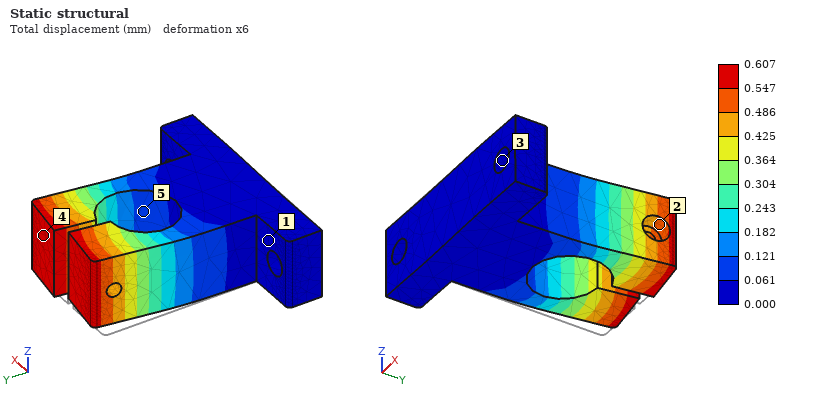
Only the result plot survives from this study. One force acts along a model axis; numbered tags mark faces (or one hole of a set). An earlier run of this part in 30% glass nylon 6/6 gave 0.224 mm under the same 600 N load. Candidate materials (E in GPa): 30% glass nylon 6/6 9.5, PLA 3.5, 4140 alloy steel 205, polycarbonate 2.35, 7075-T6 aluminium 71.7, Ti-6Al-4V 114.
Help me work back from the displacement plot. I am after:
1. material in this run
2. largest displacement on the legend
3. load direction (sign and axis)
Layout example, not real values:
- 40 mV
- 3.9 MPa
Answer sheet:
- PLA
- 0.607 mm
- +X
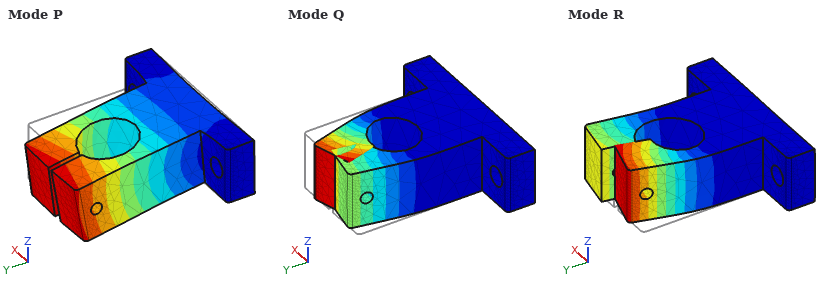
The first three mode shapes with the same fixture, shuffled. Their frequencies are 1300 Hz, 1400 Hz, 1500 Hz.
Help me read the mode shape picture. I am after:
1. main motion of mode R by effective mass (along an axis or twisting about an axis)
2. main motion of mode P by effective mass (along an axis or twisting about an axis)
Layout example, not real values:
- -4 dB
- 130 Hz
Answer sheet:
- along X
- along Z
